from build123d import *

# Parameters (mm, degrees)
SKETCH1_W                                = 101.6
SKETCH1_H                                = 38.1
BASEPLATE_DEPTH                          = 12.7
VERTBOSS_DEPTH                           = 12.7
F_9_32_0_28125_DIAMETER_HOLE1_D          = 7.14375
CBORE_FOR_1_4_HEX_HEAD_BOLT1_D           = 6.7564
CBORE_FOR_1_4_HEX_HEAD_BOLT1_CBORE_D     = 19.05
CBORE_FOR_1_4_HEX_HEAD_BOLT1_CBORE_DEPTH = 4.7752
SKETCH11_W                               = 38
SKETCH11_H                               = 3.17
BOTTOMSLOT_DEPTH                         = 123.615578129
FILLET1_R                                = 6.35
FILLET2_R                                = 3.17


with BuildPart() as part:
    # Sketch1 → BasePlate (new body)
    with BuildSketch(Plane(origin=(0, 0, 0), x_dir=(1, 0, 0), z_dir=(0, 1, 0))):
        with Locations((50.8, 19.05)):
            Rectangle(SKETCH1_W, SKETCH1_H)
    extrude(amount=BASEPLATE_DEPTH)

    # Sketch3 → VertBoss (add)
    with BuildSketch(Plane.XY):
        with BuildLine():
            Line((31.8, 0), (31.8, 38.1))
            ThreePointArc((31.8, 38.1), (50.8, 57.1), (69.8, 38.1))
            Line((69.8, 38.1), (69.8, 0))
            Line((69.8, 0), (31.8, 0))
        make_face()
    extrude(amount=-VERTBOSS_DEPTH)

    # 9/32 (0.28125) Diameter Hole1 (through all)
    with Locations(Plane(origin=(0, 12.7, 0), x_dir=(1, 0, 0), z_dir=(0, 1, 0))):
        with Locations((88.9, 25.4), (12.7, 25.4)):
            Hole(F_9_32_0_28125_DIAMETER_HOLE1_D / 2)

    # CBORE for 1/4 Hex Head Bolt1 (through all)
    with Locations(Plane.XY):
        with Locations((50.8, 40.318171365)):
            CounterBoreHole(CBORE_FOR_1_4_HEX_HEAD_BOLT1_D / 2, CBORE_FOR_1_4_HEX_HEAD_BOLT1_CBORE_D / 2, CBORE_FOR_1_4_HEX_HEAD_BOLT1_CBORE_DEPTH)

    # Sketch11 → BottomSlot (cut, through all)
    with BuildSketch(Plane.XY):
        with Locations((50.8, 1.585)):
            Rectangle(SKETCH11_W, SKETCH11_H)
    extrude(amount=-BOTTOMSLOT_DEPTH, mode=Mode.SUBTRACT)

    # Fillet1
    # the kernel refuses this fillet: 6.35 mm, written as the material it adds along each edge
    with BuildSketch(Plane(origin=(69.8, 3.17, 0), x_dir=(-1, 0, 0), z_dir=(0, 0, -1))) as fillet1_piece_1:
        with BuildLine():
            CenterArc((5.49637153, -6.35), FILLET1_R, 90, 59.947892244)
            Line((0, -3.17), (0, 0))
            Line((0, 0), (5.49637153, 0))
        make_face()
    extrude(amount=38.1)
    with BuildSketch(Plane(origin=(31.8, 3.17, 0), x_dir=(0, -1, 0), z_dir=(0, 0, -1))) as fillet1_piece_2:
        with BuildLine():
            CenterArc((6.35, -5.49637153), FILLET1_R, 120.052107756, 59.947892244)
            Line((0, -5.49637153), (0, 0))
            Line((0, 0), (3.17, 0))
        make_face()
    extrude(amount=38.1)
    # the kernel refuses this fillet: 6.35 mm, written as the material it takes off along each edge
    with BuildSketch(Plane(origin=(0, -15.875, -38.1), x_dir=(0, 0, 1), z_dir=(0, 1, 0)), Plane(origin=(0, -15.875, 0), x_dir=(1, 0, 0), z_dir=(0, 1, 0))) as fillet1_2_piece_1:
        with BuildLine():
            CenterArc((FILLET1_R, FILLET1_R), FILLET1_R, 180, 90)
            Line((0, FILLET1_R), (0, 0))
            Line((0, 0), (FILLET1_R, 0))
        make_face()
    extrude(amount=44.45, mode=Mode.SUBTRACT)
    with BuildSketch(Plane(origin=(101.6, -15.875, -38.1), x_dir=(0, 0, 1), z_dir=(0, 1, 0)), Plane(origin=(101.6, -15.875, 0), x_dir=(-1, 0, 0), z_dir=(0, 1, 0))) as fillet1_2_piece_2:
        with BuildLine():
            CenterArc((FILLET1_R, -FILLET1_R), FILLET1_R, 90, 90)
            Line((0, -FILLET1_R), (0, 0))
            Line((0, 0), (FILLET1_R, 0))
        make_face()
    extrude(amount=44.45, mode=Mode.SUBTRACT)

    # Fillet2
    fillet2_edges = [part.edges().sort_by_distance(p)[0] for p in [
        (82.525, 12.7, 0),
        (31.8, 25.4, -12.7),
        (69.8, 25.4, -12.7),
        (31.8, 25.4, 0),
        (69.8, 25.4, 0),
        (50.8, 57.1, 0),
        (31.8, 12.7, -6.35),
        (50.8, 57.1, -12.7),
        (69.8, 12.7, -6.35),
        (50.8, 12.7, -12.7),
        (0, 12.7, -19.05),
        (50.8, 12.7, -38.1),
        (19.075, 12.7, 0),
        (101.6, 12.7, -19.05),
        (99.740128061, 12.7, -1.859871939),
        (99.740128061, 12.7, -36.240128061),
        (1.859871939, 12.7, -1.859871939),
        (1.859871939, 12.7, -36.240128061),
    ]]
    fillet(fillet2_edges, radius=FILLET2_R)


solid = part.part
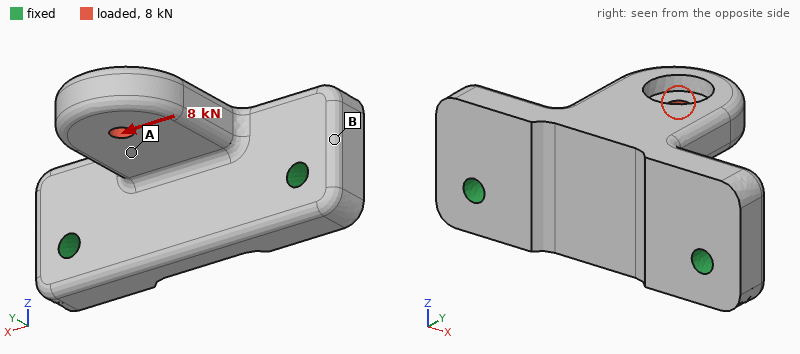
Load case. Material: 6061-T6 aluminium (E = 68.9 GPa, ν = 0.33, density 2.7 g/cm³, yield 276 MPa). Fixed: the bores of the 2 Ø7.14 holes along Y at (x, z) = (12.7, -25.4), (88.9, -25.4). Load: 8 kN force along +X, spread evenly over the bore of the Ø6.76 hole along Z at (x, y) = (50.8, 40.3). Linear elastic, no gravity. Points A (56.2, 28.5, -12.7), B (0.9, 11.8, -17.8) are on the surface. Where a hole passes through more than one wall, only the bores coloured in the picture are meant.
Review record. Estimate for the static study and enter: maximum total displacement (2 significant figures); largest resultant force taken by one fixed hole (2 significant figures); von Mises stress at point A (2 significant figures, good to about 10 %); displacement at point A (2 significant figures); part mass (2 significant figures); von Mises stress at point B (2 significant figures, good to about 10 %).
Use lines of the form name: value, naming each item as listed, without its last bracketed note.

maximum total displacement: 0.19 mm
largest resultant force taken by one fixed hole: 6.2 kN
von Mises stress at point A: 63 MPa
displacement at point A: 0.085 mm
part mass: 160 g
von Mises stress at point B: 20 MPa
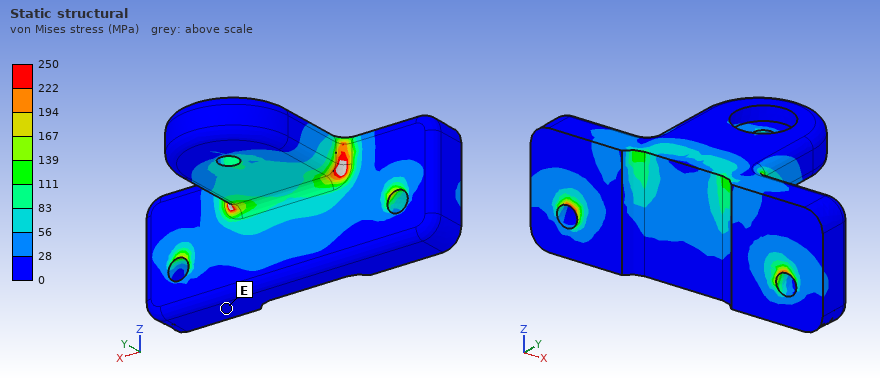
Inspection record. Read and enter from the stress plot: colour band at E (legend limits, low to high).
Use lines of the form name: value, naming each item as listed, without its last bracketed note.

colour band at E: 0 to 28 MPa
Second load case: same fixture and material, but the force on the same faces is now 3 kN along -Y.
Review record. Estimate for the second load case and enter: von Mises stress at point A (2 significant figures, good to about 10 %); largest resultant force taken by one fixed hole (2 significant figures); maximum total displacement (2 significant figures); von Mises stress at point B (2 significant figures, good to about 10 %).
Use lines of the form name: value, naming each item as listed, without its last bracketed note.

von Mises stress at point A: 14 MPa
largest resultant force taken by one fixed hole: 1.6 kN
maximum total displacement: 54 µm
von Mises stress at point B: 9.6 MPa
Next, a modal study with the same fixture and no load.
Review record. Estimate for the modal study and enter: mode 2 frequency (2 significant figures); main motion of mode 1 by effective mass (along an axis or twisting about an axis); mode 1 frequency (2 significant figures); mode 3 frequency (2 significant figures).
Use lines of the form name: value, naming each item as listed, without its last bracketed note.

mode 2 frequency: 6300 Hz
main motion of mode 1 by effective mass: along Z
mode 1 frequency: 3000 Hz
mode 3 frequency: 6600 Hz
